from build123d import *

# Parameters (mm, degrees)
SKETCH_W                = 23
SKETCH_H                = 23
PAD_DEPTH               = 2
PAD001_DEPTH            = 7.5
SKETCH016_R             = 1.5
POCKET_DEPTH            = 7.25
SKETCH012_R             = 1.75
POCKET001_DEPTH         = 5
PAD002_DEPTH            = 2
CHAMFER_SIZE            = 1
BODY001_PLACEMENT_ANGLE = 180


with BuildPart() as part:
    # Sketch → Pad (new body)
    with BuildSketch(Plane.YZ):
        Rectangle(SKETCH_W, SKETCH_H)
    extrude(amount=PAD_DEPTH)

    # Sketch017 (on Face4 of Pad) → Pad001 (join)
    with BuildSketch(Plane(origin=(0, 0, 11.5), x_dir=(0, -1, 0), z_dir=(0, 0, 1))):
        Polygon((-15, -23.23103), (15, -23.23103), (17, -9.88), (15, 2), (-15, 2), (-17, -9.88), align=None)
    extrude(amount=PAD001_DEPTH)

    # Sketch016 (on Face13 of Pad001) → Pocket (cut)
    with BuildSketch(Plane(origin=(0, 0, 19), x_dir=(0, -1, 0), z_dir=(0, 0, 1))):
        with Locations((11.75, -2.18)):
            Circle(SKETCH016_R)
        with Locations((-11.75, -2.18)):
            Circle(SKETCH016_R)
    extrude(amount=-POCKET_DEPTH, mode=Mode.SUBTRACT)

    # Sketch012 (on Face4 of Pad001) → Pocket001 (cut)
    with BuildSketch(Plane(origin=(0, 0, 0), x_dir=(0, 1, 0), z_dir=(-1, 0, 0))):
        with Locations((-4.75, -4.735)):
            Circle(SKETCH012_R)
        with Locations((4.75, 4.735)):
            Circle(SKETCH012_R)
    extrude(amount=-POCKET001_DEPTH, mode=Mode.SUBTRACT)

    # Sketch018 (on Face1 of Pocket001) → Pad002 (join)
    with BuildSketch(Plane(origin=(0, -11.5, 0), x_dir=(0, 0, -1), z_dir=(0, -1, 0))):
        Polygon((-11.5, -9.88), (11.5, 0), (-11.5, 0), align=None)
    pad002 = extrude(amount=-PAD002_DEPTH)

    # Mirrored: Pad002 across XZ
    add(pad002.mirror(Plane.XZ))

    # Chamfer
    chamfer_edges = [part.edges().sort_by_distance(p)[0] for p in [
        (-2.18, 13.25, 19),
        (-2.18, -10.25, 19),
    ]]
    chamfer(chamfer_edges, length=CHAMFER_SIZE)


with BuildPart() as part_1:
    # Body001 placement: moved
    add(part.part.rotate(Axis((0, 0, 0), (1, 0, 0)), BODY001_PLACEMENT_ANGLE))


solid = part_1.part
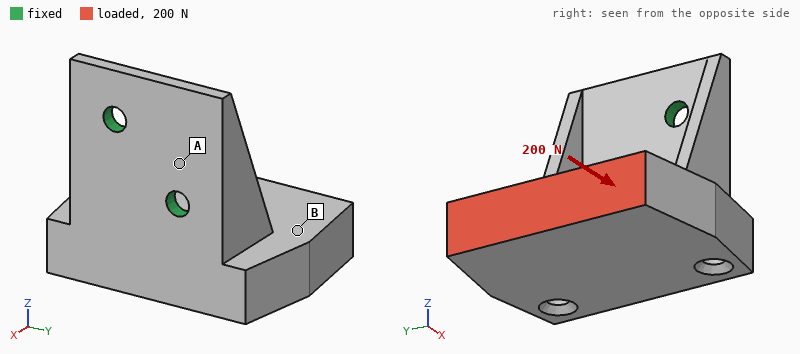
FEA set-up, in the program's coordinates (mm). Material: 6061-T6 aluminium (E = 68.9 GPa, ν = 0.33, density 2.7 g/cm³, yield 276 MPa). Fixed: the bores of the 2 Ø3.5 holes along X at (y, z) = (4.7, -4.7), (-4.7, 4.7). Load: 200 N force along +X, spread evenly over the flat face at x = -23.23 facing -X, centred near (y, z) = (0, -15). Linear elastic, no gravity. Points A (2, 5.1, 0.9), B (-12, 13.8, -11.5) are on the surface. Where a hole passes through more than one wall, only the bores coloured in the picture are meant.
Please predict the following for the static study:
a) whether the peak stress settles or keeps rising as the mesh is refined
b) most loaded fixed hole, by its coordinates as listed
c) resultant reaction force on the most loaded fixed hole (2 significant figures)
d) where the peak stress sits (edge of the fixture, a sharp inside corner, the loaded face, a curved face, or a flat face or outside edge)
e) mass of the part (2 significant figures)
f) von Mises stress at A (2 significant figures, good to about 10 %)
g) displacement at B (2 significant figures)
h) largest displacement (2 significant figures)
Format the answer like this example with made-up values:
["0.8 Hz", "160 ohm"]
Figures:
["keeps rising", "(4.7, -4.7)", "210 N", "edge of the fixture", "20 g", "22 MPa", "0.039 mm", "0.10 mm"]
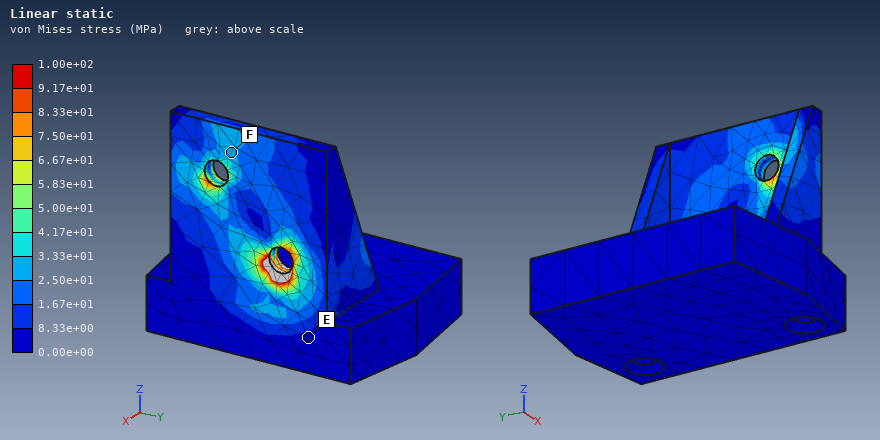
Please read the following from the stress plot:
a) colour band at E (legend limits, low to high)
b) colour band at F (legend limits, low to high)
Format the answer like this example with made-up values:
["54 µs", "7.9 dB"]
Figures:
["0.00e+00 to 8.33e+00 MPa", "2.50e+01 to 3.33e+01 MPa"]
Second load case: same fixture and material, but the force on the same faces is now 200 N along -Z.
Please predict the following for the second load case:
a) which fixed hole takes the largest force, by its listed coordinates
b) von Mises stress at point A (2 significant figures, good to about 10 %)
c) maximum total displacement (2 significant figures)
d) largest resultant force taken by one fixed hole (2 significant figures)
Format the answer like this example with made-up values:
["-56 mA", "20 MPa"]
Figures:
["(-4.7, 4.7)", "53 MPa", "0.19 mm", "210 N"]
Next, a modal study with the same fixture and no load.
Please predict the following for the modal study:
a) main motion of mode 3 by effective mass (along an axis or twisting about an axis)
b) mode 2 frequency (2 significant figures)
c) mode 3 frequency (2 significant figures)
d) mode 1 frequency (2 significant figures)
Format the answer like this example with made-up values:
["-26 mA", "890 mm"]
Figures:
["along X", "3200 Hz", "8500 Hz", "1800 Hz"]
